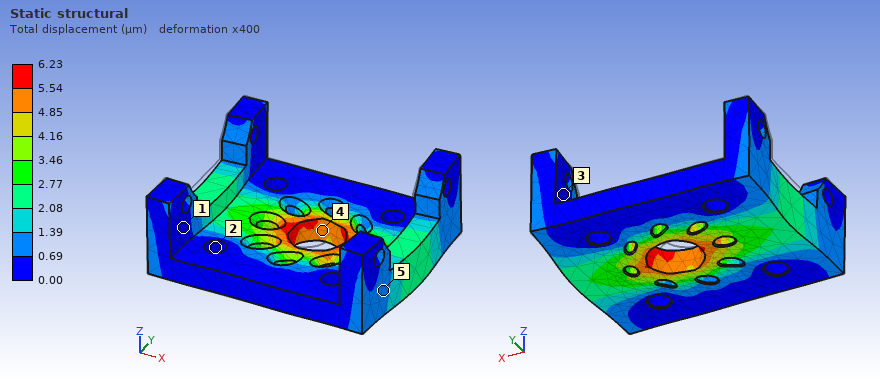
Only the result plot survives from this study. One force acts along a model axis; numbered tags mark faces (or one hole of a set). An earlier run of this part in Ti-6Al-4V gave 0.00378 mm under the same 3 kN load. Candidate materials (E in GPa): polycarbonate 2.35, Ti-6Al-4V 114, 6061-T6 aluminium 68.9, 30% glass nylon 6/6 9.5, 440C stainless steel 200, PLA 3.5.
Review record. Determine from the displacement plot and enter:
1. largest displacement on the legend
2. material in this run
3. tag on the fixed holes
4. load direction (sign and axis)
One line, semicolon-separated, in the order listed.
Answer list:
6.23 µm; 6061-T6 aluminium; 2; +X
